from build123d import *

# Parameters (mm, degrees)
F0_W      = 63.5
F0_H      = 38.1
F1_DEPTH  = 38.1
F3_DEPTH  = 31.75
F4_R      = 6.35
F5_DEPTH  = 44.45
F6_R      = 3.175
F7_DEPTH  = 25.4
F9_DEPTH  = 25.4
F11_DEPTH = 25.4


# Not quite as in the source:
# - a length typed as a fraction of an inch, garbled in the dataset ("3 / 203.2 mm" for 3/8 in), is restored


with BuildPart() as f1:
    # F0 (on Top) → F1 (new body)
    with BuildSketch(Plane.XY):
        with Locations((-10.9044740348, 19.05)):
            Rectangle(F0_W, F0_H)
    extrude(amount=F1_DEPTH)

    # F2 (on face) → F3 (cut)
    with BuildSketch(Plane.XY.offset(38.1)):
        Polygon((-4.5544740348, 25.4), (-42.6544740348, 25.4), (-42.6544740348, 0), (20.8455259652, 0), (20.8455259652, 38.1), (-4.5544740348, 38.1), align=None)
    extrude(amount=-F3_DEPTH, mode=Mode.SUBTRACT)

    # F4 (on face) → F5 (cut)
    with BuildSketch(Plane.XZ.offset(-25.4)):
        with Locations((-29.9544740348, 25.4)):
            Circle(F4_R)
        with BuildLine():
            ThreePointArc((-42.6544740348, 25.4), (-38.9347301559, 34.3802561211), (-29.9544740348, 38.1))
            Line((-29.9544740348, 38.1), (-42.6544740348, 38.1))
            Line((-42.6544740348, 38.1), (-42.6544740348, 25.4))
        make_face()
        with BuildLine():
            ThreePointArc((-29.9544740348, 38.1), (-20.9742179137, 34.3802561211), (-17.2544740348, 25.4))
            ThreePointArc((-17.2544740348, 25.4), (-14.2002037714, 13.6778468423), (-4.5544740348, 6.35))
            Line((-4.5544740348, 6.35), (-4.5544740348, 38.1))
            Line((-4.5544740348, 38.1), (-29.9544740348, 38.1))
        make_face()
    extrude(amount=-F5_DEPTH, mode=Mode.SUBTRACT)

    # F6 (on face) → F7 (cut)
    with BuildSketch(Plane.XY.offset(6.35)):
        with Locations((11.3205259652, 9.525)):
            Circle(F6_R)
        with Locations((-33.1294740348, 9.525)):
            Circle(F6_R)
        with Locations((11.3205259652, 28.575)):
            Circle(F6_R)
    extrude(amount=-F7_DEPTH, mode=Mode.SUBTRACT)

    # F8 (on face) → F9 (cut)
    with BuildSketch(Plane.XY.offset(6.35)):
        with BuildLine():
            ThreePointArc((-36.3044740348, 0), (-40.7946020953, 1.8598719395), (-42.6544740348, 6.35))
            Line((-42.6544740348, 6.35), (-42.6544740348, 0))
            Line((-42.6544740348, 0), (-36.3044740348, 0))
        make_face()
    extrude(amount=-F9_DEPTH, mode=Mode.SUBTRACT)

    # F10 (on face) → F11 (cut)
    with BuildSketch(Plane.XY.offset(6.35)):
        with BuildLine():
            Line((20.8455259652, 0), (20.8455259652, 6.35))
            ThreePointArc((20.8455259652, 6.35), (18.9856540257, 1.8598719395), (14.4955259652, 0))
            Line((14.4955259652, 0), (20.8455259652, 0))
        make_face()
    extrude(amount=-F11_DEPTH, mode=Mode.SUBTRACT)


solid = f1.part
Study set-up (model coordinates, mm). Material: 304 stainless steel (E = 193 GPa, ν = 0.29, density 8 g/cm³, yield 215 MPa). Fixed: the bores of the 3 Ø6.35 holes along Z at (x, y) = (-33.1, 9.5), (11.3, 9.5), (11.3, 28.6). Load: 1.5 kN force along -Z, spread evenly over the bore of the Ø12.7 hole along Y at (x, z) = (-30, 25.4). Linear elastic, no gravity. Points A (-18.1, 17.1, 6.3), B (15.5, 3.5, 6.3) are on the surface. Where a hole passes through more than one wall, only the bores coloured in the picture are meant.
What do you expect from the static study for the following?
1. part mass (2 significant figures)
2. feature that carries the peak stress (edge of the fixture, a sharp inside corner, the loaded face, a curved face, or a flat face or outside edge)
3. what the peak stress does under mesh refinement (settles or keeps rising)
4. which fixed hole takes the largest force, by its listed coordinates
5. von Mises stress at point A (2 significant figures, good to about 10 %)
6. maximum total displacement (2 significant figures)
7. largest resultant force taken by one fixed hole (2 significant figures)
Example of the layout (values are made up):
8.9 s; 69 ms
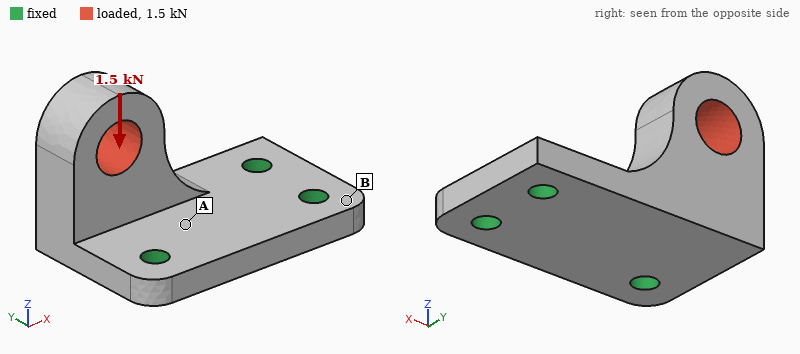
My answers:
190 g; edge of the fixture; keeps rising; (-33.1, 9.5); 32 MPa; 57 µm; 1.2 kN
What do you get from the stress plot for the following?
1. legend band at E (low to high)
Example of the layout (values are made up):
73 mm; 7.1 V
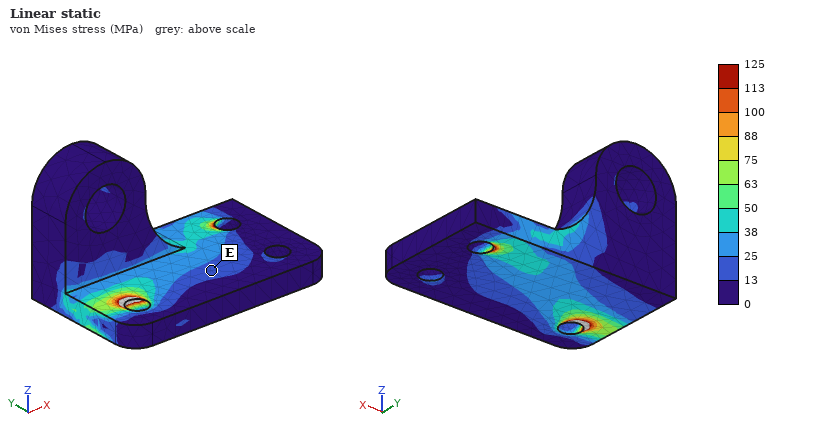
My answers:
13 to 25 MPa
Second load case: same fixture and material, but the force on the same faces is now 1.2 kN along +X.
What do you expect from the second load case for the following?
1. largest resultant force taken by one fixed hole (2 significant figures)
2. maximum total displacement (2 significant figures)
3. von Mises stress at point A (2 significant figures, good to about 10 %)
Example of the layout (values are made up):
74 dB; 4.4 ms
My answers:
770 N; 30 µm; 20 MPa
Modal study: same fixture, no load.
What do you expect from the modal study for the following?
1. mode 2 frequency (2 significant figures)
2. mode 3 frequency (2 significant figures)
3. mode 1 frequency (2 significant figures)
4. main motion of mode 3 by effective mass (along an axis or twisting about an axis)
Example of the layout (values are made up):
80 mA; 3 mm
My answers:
6500 Hz; 8800 Hz; 2900 Hz; along Z
